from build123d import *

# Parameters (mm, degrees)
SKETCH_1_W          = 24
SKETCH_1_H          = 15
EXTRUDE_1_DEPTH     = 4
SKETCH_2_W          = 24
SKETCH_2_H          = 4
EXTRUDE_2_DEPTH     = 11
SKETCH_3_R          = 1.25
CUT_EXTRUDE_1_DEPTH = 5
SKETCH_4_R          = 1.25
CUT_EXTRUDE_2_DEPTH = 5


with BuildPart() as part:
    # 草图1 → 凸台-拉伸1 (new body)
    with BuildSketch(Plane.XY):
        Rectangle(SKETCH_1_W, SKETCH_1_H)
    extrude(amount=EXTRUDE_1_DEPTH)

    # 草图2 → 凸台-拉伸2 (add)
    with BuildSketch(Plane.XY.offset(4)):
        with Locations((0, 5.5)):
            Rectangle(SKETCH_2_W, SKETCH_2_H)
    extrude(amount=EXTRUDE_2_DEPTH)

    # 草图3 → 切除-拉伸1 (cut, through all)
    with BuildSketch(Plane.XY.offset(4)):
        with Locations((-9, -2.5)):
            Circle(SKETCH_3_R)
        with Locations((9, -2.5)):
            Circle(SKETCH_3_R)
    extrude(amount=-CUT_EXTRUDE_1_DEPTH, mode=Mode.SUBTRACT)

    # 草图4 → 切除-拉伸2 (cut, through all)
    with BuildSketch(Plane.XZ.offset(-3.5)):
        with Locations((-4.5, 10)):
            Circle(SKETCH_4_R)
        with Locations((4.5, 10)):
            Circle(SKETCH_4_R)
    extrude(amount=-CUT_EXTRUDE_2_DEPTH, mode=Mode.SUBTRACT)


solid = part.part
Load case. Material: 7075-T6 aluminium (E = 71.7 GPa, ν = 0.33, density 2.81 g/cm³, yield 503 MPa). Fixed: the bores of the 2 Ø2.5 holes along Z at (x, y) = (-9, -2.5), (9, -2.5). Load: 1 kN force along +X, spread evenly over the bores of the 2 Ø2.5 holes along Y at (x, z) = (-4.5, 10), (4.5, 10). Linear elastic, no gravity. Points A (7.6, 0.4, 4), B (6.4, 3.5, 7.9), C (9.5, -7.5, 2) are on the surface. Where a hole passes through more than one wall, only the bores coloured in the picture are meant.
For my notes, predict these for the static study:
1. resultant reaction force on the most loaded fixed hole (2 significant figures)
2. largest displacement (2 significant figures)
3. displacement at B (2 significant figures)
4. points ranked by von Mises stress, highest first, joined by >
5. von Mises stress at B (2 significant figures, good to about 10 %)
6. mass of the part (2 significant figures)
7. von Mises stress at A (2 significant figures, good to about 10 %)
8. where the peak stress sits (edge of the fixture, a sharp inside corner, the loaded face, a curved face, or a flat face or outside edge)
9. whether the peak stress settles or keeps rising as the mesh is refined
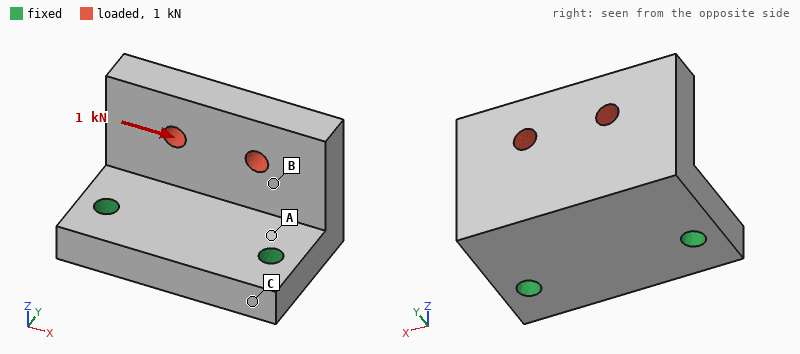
770 N
32 µm
16 µm
A > B > C
29 MPa
6.8 g
55 MPa
edge of the fixture
keeps rising
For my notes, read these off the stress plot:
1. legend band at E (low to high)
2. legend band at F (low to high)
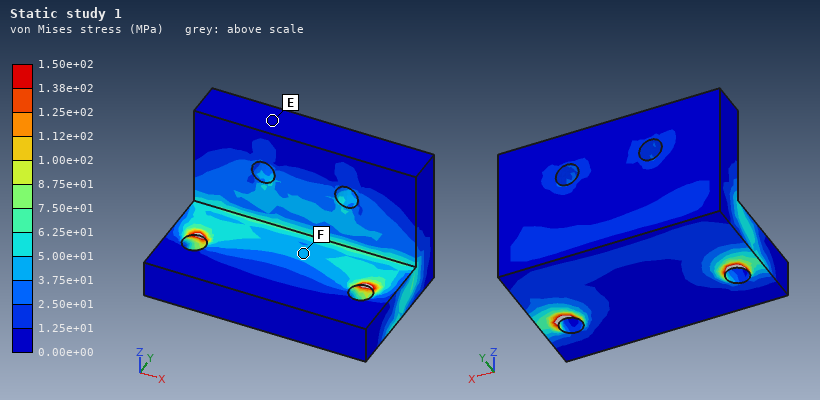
0.00e+00 to 1.25e+01 MPa
3.75e+01 to 5.00e+01 MPa
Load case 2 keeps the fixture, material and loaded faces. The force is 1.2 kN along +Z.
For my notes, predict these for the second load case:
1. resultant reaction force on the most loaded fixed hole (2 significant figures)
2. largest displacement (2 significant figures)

600 N
80 µm
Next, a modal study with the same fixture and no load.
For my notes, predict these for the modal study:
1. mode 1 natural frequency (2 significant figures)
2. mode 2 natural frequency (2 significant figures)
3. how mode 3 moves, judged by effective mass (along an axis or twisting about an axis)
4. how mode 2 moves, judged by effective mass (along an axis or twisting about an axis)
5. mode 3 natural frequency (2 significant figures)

9200 Hz
17 kHz
along Z
along X
25 kHz
